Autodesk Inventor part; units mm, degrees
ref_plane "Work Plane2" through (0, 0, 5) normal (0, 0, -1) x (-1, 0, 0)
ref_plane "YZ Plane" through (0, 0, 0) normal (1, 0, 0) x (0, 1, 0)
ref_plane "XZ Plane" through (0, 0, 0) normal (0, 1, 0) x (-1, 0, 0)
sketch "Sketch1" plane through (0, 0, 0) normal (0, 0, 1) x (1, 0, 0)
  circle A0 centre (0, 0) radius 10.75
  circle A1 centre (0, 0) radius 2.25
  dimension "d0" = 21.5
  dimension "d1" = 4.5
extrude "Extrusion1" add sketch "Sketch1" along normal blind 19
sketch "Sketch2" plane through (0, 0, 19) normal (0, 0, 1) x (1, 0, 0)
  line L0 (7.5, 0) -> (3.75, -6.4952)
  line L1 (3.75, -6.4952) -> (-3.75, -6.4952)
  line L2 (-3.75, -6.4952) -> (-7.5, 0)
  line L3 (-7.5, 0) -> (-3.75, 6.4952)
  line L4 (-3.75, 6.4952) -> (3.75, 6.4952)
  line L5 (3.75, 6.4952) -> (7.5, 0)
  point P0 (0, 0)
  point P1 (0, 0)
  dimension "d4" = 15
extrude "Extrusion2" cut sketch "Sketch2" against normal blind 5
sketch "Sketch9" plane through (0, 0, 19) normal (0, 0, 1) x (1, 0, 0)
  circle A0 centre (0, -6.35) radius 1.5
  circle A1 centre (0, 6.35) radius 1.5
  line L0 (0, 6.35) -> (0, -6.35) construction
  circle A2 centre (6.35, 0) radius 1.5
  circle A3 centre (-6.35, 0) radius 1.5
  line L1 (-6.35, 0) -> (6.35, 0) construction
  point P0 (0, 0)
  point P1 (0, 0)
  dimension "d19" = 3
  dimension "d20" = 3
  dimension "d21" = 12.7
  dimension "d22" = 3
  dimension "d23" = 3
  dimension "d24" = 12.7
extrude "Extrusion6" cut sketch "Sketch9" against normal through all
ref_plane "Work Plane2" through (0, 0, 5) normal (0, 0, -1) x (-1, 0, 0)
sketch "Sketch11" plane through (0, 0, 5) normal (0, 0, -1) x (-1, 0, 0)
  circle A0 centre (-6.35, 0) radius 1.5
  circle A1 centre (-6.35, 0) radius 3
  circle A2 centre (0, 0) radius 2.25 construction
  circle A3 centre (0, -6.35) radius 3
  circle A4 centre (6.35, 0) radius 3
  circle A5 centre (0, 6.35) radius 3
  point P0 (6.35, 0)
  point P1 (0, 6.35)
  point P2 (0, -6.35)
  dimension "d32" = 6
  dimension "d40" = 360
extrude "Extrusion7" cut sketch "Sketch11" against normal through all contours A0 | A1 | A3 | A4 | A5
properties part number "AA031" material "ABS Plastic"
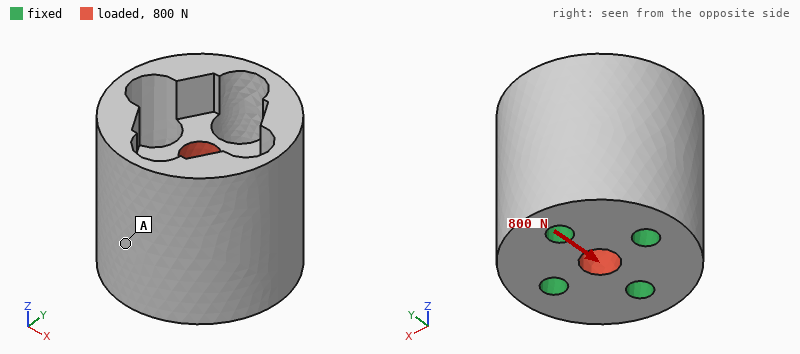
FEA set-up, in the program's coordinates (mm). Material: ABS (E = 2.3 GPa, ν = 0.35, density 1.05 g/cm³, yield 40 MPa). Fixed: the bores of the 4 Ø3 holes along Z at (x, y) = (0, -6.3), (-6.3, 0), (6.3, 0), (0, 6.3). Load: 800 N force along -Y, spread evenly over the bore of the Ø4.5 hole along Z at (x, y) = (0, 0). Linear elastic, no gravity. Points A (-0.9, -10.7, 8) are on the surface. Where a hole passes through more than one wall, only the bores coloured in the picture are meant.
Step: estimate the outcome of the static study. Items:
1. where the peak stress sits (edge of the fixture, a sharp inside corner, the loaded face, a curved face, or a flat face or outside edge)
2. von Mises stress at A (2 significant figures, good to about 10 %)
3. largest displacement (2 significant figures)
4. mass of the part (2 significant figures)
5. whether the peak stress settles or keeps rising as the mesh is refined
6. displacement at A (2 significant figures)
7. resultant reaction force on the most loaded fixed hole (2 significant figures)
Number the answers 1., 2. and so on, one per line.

1. edge of the fixture
2. 2.4 MPa
3. 79 µm
4. 4.8 g
5. keeps rising
6. 31 µm
7. 290 N
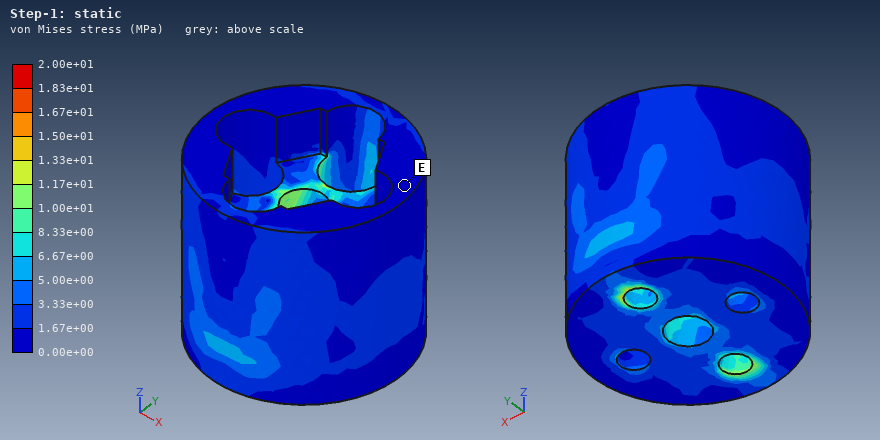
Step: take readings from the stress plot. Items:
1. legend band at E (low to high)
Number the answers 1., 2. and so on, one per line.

1. 0.00e+00 to 1.67e+00 MPa
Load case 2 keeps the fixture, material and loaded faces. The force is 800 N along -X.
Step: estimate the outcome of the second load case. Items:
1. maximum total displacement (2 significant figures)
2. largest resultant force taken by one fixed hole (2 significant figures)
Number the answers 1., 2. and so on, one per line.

1. 78 µm
2. 290 N
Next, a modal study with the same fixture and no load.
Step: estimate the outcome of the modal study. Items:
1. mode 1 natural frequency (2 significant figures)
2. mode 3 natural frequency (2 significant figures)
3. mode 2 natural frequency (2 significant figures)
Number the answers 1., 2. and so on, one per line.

1. 7700 Hz
2. 10 kHz
3. 7700 Hz
